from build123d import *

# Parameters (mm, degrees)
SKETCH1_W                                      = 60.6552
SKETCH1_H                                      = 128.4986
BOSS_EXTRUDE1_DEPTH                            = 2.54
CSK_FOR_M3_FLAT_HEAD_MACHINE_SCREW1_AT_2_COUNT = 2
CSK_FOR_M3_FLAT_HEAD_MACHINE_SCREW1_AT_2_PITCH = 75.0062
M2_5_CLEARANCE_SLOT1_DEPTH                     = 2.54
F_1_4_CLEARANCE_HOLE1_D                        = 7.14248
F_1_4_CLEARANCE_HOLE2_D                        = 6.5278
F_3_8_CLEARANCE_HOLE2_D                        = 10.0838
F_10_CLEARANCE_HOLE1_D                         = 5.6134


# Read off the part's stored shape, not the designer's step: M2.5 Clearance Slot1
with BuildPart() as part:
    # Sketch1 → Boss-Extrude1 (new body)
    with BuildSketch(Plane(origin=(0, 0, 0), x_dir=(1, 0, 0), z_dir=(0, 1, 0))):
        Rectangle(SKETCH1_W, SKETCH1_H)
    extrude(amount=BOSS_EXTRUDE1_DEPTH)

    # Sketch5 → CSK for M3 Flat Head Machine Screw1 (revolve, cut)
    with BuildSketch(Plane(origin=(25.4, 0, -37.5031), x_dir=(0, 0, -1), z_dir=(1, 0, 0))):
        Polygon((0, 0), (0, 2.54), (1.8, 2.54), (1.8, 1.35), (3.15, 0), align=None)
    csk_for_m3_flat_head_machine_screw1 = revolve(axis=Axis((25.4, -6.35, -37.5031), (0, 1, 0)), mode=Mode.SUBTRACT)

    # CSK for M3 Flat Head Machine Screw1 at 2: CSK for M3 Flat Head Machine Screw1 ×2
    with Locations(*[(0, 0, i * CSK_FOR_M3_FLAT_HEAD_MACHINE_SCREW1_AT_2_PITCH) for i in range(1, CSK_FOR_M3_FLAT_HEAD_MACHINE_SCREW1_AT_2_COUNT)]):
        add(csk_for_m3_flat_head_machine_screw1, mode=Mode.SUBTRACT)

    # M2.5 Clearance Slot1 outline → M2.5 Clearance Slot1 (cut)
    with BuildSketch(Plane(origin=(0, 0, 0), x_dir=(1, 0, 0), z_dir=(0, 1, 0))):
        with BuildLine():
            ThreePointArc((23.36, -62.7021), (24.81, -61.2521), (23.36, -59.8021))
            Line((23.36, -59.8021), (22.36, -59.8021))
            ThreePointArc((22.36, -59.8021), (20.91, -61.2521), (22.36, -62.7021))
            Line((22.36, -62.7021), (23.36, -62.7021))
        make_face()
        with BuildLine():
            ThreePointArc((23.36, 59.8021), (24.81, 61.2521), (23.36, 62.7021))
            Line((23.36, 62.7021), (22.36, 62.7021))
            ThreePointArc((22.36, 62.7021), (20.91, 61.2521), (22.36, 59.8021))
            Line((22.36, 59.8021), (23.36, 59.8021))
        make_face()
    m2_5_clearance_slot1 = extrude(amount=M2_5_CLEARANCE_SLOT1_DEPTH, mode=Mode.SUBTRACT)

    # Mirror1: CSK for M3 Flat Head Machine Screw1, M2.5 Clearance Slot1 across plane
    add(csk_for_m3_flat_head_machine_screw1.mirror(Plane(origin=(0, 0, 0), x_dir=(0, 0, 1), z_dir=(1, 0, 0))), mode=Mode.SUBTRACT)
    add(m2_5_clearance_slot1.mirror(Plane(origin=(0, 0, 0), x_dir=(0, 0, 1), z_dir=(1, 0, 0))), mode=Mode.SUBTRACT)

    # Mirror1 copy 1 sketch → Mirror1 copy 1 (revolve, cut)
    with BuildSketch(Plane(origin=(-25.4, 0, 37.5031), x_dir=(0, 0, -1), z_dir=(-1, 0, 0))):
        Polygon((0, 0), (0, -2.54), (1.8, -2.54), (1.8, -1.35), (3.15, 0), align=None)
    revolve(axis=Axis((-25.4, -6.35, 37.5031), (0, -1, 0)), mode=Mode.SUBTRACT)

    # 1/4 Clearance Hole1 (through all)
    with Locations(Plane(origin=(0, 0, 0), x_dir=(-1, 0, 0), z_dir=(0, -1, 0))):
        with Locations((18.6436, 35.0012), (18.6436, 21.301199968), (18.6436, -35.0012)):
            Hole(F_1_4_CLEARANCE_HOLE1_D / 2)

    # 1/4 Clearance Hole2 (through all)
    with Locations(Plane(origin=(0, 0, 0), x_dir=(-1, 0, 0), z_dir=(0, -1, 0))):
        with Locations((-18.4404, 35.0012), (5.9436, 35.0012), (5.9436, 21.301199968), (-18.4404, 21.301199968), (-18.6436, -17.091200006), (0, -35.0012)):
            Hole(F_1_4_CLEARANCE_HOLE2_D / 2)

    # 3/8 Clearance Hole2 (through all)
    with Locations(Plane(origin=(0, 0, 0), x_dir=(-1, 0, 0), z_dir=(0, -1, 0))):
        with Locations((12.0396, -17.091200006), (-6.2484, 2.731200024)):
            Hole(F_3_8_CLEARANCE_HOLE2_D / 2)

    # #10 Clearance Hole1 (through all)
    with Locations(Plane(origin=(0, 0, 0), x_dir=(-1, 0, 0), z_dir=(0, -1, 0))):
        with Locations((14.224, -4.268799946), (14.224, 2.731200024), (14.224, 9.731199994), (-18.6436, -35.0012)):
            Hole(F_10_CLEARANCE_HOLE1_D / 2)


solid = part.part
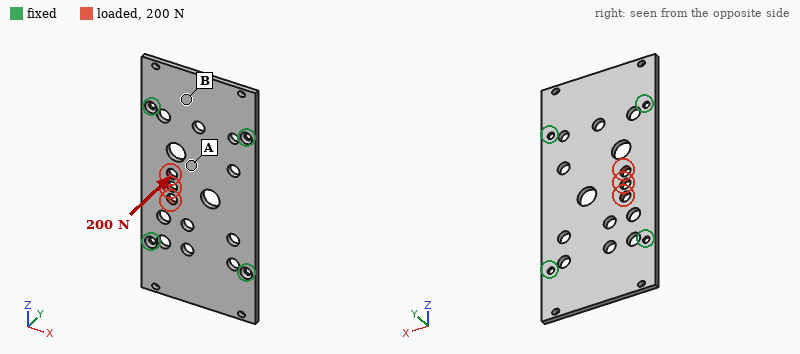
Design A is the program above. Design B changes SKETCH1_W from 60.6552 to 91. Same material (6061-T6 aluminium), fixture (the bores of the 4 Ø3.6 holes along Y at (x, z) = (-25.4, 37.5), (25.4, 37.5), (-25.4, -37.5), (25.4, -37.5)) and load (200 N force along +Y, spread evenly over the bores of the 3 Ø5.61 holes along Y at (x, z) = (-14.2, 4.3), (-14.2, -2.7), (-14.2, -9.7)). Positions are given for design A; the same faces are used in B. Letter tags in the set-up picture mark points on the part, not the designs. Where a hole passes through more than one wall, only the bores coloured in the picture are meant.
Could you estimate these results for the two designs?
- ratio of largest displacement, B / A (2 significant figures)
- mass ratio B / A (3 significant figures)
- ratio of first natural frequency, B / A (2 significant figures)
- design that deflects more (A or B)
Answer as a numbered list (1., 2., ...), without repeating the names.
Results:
1. 0.79
2. 1.55
3. 0.95
4. A
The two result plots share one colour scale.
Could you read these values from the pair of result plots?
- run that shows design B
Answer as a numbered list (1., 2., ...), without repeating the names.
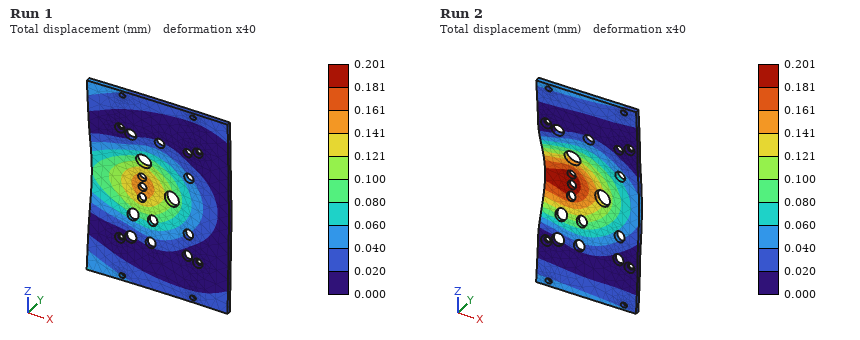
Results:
1. Run 1
